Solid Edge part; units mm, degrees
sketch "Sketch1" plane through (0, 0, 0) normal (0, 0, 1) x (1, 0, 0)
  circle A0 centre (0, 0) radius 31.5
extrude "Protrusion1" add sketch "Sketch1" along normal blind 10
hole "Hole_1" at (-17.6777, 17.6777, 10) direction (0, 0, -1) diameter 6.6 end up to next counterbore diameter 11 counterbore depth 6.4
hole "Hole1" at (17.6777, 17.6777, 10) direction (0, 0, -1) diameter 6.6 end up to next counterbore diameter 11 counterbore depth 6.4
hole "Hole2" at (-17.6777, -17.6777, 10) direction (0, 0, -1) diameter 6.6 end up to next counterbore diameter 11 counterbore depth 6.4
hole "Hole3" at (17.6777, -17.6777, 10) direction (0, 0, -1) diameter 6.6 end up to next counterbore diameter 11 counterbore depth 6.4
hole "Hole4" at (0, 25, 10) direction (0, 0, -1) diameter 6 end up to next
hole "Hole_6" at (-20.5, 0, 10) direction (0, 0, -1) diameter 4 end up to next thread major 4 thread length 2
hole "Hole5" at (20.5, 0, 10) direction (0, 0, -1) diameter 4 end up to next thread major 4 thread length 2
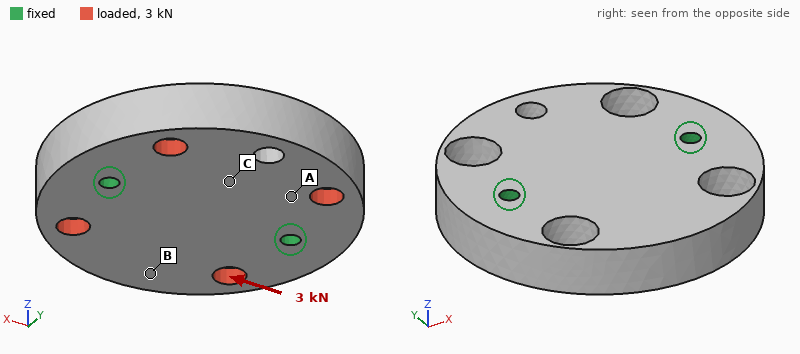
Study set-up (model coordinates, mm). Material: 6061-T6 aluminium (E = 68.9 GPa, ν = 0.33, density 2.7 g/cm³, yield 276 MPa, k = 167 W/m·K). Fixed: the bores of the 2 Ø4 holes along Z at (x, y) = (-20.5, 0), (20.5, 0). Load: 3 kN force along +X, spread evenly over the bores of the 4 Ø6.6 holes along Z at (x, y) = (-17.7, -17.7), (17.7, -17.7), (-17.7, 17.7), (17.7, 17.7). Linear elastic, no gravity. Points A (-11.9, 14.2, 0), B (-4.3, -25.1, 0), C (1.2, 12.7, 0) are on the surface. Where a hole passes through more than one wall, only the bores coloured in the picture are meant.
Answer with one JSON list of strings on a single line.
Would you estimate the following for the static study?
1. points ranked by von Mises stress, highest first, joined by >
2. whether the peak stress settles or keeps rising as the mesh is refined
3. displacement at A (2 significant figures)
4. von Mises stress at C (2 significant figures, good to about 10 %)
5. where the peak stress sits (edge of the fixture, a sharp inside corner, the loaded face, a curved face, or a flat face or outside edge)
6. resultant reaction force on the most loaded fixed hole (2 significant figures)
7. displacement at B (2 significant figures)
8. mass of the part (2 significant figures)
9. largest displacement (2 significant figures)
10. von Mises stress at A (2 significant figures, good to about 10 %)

["A > C > B", "keeps rising", "2.6 µm", "6.0 MPa", "edge of the fixture", "1.5 kN", "3.4 µm", "75 g", "5.4 µm", "9.7 MPa"]
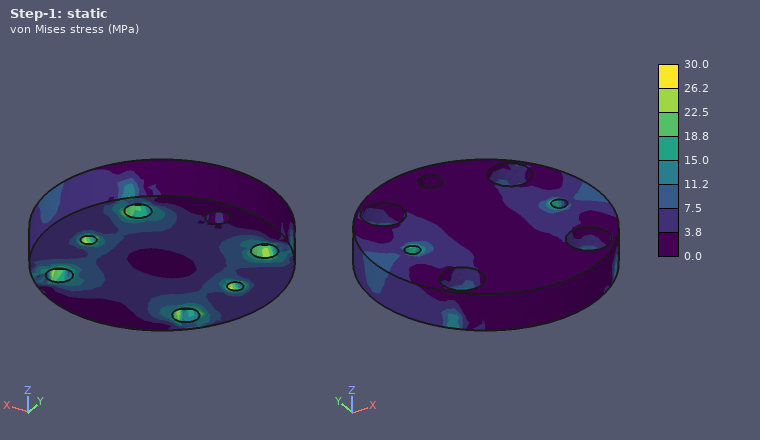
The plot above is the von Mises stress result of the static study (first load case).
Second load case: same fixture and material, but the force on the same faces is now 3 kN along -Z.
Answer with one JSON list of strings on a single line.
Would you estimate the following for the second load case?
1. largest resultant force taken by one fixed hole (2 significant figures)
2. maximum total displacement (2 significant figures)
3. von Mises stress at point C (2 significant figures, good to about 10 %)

["1.5 kN", "21 µm", "8.9 MPa"]
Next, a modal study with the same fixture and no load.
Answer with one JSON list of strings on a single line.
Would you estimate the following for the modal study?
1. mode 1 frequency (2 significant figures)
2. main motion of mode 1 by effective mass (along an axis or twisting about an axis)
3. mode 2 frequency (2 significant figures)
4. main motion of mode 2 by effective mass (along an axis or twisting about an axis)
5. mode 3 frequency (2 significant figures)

["6600 Hz", "twisting about X", "9100 Hz", "along Z", "17 kHz"]
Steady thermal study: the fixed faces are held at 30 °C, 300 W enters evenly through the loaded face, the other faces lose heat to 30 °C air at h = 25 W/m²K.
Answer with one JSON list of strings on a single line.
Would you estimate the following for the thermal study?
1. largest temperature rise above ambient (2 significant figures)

["69 K"]
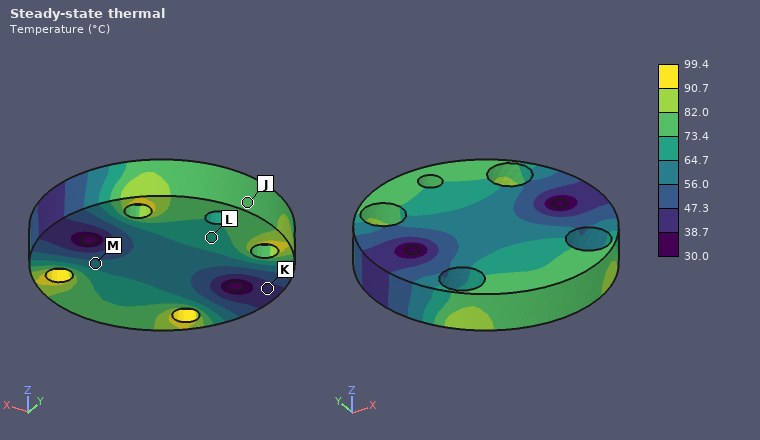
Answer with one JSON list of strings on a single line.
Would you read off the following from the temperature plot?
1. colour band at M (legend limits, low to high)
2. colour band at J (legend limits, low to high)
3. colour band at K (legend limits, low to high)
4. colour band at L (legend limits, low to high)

["56.0 to 64.7 °C", "73.4 to 82.0 °C", "38.7 to 47.3 °C", "64.7 to 73.4 °C"]
